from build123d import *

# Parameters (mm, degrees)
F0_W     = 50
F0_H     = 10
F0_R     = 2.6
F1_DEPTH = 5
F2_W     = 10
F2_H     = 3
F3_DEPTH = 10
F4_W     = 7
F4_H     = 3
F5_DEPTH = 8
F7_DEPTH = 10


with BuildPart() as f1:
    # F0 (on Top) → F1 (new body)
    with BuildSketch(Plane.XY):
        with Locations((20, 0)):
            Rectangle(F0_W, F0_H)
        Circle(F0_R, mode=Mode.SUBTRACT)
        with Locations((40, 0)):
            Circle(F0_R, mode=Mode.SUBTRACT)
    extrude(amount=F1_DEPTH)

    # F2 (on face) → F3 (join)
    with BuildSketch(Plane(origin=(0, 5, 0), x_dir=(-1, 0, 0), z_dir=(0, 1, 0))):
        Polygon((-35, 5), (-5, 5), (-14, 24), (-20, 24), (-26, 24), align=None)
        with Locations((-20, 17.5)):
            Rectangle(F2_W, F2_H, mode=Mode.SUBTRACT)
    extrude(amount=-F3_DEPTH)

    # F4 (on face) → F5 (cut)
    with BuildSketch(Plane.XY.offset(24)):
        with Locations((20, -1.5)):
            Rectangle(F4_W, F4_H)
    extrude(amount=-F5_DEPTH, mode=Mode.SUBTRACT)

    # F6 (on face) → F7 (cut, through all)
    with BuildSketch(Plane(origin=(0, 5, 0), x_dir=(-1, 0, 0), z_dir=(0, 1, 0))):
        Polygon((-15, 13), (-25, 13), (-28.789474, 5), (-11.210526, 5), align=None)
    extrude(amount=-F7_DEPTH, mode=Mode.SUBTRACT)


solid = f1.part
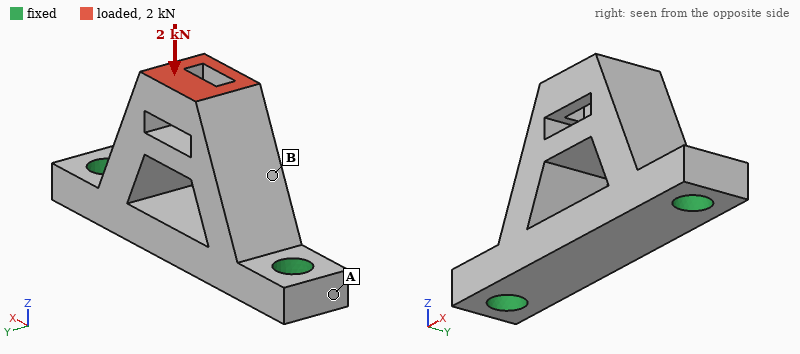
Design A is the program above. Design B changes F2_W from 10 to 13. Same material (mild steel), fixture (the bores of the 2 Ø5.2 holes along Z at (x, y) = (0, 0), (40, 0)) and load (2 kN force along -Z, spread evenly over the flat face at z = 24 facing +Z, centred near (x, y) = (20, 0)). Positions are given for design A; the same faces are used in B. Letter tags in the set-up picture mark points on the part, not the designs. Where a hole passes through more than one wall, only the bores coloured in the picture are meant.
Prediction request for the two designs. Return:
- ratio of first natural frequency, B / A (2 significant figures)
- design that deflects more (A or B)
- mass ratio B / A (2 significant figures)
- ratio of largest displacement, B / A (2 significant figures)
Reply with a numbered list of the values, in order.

1. 1.0
2. B
3. 0.98
4. 1.3
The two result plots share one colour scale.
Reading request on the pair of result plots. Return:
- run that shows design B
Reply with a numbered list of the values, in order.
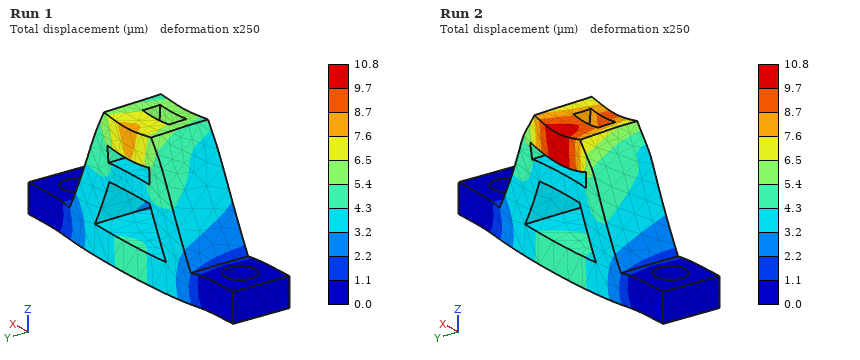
1. Run 2
